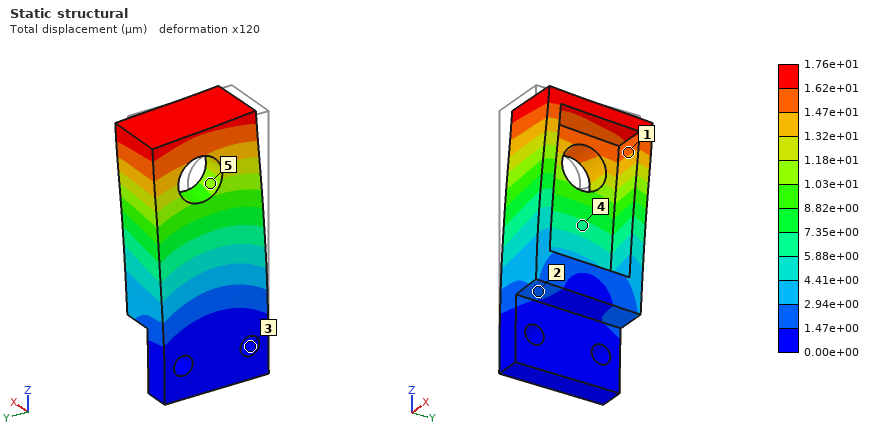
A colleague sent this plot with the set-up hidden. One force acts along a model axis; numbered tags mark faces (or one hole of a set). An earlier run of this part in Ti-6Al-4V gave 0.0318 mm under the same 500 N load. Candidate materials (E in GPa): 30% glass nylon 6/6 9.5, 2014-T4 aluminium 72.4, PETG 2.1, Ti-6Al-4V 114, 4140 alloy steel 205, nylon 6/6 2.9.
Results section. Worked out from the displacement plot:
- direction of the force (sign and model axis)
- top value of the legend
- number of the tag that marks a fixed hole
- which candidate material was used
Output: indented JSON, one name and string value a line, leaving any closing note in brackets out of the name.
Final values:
{
  "direction of the force": "+Y",
  "top value of the legend": "1.76e+01 µm",
  "number of the tag that marks a fixed hole": "3",
  "which candidate material was used": "4140 alloy steel"
}
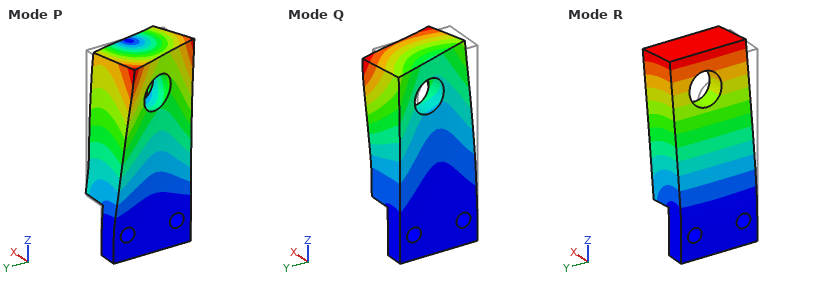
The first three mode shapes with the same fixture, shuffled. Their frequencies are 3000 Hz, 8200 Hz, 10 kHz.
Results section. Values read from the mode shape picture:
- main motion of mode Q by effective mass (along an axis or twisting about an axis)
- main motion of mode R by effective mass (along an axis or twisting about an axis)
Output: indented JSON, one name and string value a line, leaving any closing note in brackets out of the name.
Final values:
{
  "main motion of mode Q by effective mass": "along Y",
  "main motion of mode R by effective mass": "along X"
}
